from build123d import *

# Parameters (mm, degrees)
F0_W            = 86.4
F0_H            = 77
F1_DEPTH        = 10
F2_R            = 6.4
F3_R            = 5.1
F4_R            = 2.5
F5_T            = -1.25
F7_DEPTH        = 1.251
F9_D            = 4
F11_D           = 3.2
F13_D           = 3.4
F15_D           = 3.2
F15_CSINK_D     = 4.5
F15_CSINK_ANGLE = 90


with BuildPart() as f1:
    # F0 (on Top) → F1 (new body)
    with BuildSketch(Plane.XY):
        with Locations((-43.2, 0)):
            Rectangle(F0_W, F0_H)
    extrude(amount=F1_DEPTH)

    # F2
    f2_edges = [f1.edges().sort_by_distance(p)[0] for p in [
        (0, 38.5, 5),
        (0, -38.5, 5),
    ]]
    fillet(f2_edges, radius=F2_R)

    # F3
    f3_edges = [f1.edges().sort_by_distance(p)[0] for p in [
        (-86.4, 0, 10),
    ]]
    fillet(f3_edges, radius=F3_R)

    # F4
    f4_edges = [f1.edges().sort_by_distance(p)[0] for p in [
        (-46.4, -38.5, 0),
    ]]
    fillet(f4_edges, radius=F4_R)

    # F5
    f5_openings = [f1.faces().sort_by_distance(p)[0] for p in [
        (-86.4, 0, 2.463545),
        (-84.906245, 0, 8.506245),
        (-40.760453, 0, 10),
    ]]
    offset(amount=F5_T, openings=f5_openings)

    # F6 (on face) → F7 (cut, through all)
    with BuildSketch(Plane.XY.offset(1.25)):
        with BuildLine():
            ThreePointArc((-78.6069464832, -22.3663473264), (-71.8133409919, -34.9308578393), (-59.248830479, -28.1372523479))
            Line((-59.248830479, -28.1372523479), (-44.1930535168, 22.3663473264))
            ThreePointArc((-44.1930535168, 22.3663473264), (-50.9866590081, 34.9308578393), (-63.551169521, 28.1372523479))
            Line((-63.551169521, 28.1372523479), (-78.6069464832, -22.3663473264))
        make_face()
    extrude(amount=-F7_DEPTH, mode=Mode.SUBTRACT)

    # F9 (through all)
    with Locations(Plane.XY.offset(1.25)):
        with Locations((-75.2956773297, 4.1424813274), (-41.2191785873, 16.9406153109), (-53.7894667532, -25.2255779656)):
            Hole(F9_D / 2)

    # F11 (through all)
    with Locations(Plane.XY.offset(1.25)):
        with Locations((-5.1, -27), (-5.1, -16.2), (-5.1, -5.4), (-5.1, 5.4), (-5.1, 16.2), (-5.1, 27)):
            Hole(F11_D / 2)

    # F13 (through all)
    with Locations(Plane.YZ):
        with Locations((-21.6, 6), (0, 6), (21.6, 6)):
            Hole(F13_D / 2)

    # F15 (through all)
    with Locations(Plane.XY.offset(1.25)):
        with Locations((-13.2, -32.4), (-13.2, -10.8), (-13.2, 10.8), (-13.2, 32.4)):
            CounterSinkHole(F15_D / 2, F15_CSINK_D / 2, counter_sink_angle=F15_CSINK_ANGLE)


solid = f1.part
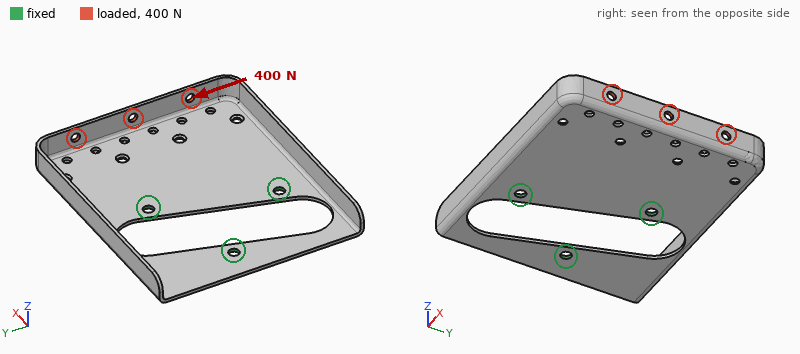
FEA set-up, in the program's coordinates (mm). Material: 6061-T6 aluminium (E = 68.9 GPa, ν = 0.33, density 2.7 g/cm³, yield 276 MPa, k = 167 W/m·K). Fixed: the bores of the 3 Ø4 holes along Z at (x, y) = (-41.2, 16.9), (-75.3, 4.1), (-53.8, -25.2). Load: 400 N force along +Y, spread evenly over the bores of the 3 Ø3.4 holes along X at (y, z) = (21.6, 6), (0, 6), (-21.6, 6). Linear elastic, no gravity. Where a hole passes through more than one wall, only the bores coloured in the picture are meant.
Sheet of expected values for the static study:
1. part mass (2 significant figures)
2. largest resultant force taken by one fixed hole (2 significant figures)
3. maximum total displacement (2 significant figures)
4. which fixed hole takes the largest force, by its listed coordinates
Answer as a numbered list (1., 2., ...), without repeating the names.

1. 24 g
2. 480 N
3. 1.2 mm
4. (-41.2, 16.9)
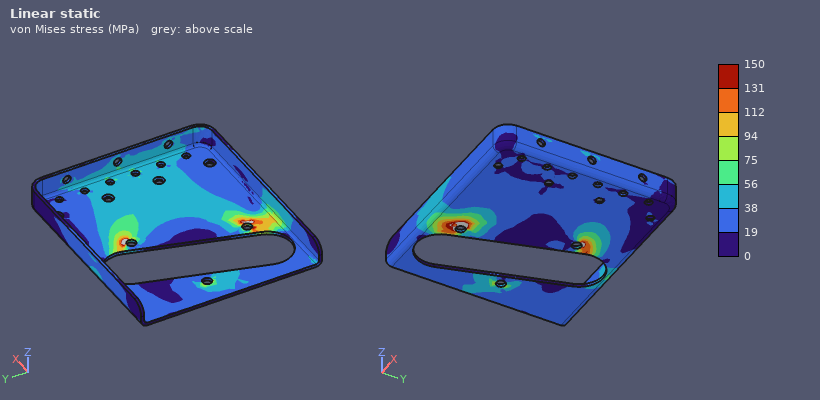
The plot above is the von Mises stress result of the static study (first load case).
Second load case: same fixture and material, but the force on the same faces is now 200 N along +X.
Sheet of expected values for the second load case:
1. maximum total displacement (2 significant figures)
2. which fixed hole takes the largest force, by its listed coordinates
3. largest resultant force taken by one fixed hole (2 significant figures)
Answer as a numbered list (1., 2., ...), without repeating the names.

1. 0.52 mm
2. (-41.2, 16.9)
3. 100 N
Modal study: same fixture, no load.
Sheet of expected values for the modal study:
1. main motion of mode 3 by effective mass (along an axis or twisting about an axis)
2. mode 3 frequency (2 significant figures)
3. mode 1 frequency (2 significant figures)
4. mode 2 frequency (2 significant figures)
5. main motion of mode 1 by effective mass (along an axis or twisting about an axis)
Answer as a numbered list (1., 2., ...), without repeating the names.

1. along Z
2. 840 Hz
3. 470 Hz
4. 680 Hz
5. along Z
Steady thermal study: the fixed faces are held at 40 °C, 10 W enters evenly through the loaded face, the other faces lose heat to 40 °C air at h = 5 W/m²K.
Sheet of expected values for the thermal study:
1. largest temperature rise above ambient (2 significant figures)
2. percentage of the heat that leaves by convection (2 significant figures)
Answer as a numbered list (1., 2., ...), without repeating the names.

1. 38 K
2. 9.7 %
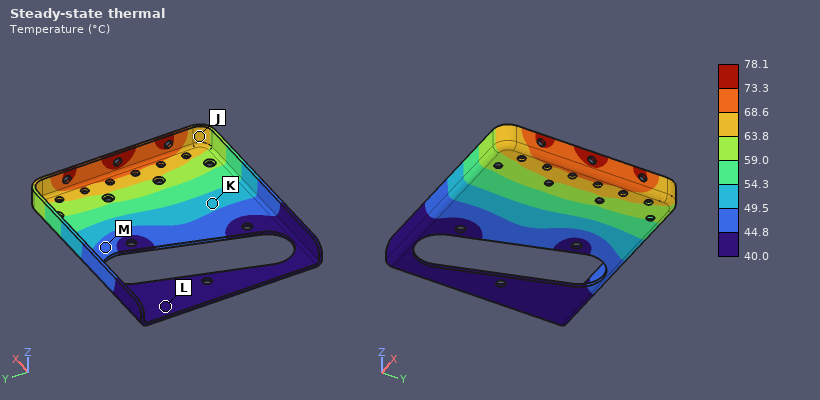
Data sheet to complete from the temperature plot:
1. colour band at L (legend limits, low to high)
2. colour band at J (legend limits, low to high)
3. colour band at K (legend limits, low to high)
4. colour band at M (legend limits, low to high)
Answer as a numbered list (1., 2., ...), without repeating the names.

1. 40.0 to 44.8 °C
2. 63.8 to 68.6 °C
3. 49.5 to 54.3 °C
4. 44.8 to 49.5 °C
